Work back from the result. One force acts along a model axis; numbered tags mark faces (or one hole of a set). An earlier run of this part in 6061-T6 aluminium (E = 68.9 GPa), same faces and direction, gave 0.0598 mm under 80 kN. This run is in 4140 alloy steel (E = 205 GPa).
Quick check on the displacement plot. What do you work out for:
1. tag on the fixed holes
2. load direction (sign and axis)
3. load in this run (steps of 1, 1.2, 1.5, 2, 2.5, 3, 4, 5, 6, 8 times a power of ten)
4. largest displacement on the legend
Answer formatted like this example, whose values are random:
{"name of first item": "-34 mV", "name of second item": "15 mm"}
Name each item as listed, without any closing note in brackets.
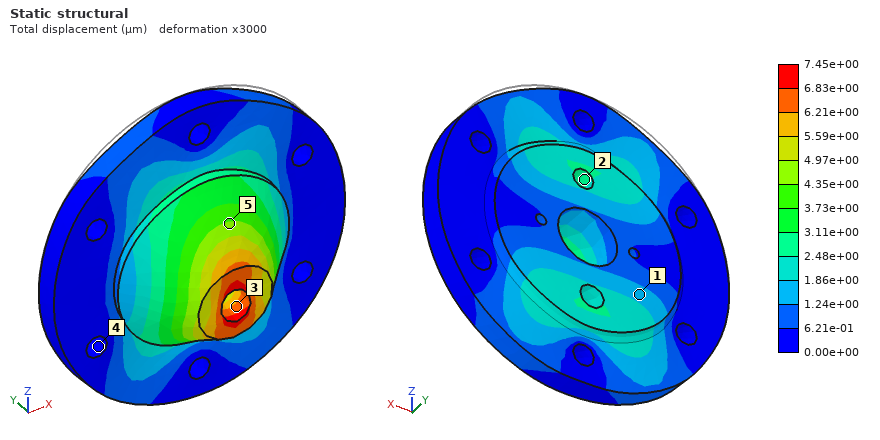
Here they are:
{"tag on the fixed holes": "4", "load direction": "-Z", "load in this run": "30 kN", "largest displacement on the legend": "7.45e+00 µm"}
